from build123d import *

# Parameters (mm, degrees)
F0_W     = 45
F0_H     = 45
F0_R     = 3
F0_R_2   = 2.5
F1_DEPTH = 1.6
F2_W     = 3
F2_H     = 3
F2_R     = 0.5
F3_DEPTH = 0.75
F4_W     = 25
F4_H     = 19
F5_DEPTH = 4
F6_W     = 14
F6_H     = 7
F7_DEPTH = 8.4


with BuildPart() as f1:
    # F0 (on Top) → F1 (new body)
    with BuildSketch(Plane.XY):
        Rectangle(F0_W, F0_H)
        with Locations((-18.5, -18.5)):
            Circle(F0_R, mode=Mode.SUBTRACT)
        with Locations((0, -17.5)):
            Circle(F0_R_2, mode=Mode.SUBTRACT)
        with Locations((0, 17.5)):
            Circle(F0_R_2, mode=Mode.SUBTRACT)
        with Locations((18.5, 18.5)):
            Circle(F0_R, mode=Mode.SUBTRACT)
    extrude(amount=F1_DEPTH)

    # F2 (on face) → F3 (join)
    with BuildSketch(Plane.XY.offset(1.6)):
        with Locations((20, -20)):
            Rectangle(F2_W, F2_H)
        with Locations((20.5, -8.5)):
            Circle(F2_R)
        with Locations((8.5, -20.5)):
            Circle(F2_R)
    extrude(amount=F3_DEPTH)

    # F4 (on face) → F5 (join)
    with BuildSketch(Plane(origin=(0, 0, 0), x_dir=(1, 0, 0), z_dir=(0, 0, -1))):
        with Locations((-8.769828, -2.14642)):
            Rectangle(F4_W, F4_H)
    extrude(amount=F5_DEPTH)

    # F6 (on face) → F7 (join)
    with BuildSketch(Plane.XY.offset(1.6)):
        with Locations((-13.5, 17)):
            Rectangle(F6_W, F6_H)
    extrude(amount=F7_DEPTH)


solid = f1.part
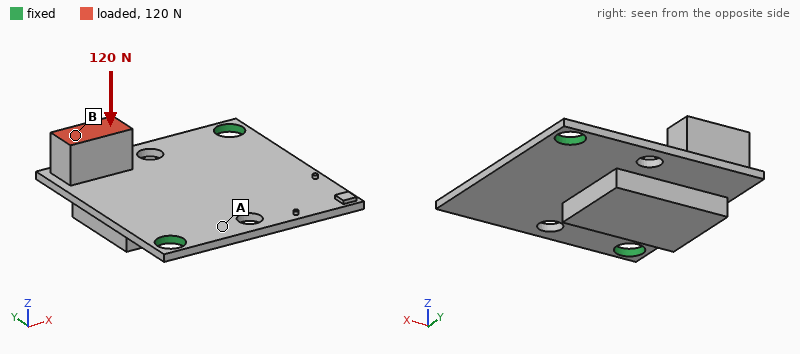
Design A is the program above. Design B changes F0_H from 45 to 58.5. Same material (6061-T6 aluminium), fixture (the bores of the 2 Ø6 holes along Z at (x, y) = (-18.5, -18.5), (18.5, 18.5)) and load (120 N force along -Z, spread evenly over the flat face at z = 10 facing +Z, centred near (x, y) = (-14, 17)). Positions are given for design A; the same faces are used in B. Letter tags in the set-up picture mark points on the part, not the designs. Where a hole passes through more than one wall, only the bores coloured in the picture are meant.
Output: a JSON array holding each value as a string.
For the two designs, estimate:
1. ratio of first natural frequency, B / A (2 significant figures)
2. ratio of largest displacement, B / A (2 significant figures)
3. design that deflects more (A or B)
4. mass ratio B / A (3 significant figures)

["0.98", "0.91", "A", "1.17"]
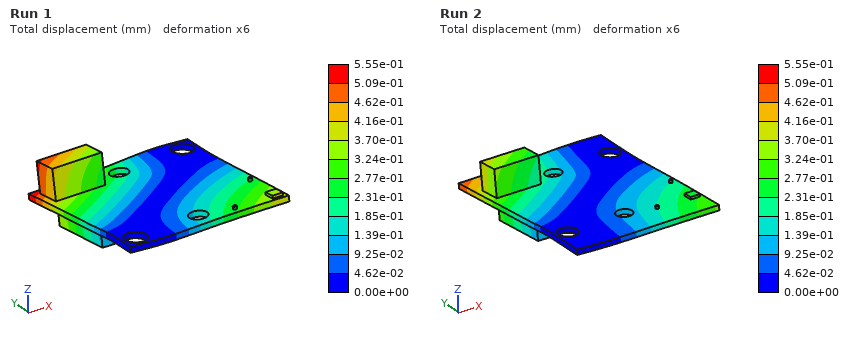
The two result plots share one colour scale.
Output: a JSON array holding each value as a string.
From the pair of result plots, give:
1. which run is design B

["Run 2"]
